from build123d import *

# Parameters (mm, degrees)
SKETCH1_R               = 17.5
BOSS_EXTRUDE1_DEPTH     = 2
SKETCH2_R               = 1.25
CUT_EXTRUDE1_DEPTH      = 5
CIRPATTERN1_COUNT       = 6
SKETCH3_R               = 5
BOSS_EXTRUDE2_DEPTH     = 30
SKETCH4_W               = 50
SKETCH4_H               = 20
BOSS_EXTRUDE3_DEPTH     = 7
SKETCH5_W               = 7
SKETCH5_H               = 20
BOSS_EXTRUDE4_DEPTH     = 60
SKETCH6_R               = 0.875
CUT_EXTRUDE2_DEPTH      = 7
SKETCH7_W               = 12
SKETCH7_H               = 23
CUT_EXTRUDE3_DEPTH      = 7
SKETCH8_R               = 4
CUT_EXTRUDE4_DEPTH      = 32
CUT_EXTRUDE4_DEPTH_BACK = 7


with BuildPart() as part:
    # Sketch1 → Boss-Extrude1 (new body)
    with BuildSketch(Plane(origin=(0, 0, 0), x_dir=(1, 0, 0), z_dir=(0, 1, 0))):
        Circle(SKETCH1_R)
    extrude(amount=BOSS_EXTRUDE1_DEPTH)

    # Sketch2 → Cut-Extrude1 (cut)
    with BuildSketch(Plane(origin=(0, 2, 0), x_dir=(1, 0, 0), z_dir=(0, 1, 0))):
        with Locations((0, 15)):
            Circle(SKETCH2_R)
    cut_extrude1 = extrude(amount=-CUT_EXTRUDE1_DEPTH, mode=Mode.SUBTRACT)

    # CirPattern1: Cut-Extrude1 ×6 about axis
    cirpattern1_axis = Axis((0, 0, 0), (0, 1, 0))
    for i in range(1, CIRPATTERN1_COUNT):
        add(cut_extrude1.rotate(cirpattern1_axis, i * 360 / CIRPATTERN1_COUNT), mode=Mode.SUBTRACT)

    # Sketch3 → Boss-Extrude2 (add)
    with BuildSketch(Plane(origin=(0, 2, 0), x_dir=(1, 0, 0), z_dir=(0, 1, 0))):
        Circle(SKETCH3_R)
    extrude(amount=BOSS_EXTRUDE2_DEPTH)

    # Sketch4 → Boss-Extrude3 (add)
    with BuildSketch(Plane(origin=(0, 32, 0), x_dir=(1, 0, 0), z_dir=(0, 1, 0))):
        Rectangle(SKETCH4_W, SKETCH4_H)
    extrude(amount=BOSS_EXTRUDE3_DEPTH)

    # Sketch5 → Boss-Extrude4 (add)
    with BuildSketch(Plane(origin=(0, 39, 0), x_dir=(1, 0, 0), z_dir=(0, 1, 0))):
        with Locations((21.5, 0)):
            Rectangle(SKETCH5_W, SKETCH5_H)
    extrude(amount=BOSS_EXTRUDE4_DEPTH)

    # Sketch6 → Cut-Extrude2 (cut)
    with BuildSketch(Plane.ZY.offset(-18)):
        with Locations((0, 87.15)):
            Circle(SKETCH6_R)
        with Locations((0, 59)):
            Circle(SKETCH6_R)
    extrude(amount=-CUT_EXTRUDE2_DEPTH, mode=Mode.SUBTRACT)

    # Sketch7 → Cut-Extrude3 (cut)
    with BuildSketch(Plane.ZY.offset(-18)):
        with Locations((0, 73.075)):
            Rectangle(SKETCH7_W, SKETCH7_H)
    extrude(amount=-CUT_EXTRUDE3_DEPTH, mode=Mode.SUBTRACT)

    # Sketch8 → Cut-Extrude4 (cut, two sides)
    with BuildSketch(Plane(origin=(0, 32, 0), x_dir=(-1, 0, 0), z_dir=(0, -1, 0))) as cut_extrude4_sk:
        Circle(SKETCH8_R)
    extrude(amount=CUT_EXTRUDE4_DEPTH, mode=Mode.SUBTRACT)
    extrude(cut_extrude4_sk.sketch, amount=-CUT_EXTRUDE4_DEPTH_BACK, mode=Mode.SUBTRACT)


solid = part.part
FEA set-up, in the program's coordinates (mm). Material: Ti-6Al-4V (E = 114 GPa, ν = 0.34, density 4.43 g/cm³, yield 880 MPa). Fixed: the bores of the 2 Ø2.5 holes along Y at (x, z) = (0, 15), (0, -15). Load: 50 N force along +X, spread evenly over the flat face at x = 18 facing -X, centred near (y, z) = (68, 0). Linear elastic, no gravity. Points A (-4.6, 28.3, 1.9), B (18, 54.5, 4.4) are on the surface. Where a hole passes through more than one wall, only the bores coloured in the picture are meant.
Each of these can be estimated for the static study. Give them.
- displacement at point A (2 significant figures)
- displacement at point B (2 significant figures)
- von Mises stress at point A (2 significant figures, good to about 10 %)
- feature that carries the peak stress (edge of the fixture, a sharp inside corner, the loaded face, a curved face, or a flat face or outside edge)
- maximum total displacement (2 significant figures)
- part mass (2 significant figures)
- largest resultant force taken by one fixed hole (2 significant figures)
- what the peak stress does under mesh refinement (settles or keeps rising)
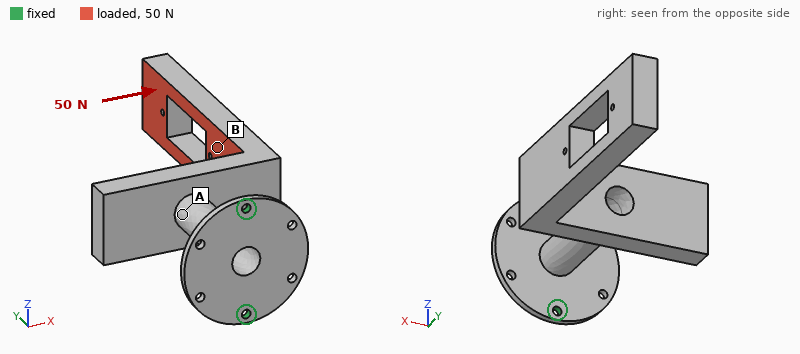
0.29 mm
0.65 mm
29 MPa
edge of the fixture
1.2 mm
70 g
25 N
keeps rising
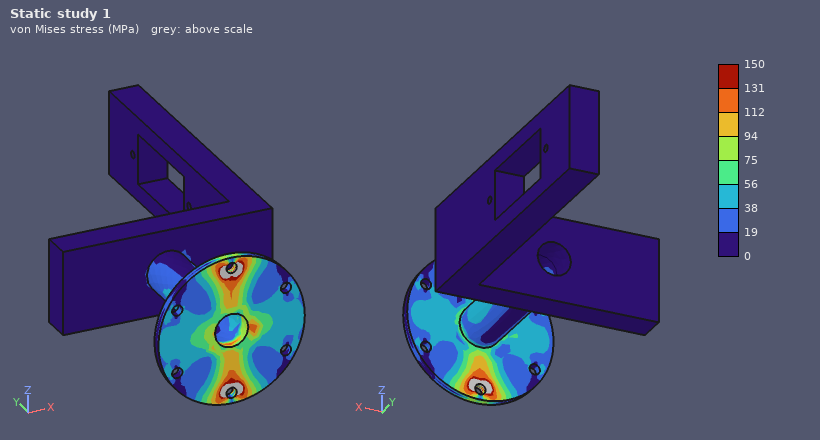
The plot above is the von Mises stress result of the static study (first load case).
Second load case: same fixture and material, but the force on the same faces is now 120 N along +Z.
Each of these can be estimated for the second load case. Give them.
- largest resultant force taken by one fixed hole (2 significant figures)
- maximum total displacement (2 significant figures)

370 N
1.3 mm
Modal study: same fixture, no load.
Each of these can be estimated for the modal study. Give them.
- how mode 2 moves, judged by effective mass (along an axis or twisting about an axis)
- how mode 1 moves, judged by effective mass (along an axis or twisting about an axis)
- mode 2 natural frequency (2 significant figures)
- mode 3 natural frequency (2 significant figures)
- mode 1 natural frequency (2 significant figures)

along Z
along X
310 Hz
1300 Hz
190 Hz
